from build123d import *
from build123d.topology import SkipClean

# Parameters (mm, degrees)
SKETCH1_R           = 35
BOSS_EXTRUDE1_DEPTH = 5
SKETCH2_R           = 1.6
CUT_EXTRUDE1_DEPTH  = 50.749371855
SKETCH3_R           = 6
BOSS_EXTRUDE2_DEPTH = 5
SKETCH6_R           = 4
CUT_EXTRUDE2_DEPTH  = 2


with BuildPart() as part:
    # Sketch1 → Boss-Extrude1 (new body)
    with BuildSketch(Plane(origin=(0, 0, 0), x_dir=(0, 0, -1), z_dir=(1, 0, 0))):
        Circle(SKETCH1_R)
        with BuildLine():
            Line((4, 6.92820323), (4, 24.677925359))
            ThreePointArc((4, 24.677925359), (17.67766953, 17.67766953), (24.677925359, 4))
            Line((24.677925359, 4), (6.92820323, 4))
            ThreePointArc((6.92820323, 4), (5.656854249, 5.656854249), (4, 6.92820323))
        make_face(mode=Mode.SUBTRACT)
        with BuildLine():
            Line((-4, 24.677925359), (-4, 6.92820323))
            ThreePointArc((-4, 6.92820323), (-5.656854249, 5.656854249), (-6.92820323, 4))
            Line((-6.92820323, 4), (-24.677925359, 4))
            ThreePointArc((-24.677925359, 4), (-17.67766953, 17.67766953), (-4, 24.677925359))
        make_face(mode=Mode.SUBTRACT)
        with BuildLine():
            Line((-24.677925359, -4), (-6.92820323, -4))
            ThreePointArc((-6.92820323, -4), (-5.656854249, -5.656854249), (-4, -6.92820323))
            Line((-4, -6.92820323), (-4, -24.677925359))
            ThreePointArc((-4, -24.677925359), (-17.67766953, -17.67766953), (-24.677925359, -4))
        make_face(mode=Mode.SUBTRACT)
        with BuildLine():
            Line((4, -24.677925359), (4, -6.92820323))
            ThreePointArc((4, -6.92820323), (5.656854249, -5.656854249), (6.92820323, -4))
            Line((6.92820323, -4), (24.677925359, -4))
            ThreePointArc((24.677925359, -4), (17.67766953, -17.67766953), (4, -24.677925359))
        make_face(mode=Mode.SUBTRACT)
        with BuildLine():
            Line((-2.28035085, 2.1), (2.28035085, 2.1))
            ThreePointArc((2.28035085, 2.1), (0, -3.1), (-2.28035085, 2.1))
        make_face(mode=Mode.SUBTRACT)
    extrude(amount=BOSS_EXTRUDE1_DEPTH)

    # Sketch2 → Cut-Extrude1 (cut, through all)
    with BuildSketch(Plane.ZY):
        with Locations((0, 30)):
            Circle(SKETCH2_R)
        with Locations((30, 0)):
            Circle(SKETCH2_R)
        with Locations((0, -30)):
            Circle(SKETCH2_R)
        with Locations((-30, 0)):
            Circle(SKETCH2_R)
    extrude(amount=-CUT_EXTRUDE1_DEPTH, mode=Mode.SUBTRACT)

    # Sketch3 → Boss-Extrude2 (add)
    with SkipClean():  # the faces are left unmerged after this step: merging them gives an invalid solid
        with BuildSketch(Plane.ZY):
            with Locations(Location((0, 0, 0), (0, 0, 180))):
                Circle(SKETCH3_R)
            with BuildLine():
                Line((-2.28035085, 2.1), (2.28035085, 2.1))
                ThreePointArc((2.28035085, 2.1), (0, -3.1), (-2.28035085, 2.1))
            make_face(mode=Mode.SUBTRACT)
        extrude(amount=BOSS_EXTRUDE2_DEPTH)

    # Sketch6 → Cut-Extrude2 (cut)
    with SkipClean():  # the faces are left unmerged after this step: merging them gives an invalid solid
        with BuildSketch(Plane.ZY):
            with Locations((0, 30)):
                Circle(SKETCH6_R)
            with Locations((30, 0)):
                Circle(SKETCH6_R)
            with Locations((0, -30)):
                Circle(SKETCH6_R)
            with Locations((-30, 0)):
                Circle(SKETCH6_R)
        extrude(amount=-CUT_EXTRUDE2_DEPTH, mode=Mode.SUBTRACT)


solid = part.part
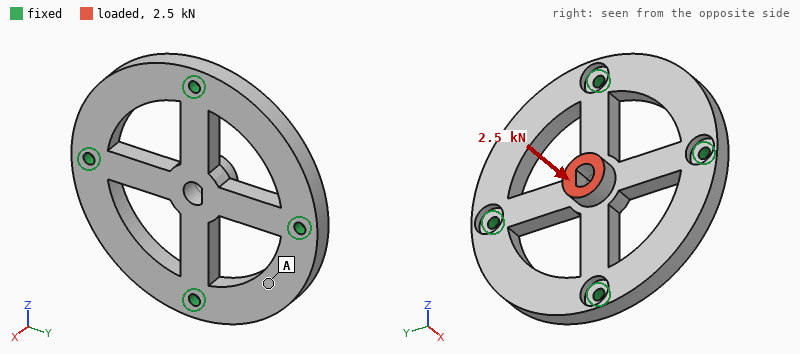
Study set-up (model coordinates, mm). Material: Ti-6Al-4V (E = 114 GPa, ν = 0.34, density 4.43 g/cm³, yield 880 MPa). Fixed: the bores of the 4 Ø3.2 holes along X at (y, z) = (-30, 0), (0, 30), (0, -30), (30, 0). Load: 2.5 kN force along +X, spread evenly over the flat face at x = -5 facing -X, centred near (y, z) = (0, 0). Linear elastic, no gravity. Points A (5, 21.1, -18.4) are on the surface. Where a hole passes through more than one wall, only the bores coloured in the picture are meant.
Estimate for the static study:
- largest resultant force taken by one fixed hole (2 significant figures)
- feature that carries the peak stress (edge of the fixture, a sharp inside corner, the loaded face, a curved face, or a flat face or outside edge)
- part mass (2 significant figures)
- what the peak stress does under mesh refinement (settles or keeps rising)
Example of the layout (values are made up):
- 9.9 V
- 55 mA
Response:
- 1.1 kN
- edge of the fixture
- 58 g
- keeps rising
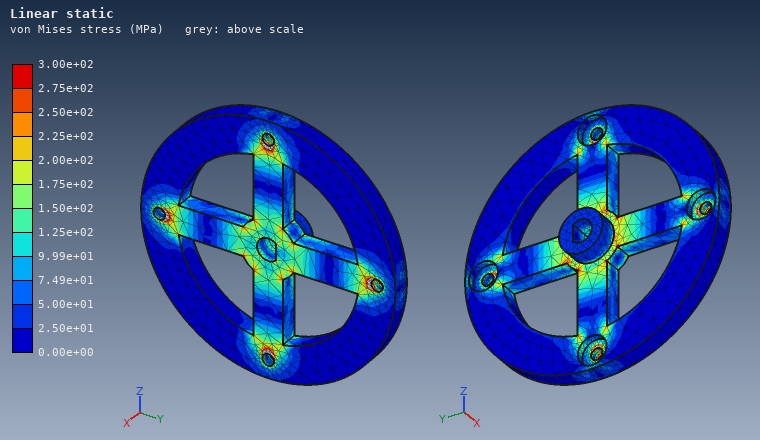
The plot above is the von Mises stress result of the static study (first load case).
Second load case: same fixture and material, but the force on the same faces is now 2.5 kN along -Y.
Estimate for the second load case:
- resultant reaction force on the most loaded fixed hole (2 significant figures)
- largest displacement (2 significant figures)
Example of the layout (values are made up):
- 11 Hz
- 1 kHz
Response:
- 1.2 kN
- 49 µm
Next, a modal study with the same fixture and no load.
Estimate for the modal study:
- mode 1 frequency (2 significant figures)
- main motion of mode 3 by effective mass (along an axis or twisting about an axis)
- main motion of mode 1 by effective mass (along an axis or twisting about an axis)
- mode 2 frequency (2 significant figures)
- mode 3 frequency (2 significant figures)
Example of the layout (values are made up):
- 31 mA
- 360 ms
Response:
- 7000 Hz
- twisting about Y
- along X
- 7500 Hz
- 8300 Hz
